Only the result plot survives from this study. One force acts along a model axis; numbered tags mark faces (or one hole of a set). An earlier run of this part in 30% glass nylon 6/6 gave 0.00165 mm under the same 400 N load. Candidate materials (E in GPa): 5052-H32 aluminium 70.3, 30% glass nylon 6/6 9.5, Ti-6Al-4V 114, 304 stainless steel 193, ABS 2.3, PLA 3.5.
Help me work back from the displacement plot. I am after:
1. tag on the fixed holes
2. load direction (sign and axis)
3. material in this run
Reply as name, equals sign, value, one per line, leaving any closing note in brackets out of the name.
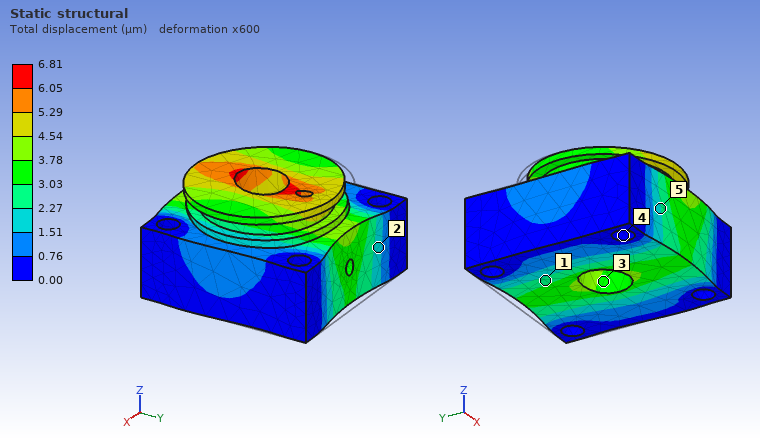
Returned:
tag on the fixed holes = 4
load direction = -Y
material in this run = ABS
